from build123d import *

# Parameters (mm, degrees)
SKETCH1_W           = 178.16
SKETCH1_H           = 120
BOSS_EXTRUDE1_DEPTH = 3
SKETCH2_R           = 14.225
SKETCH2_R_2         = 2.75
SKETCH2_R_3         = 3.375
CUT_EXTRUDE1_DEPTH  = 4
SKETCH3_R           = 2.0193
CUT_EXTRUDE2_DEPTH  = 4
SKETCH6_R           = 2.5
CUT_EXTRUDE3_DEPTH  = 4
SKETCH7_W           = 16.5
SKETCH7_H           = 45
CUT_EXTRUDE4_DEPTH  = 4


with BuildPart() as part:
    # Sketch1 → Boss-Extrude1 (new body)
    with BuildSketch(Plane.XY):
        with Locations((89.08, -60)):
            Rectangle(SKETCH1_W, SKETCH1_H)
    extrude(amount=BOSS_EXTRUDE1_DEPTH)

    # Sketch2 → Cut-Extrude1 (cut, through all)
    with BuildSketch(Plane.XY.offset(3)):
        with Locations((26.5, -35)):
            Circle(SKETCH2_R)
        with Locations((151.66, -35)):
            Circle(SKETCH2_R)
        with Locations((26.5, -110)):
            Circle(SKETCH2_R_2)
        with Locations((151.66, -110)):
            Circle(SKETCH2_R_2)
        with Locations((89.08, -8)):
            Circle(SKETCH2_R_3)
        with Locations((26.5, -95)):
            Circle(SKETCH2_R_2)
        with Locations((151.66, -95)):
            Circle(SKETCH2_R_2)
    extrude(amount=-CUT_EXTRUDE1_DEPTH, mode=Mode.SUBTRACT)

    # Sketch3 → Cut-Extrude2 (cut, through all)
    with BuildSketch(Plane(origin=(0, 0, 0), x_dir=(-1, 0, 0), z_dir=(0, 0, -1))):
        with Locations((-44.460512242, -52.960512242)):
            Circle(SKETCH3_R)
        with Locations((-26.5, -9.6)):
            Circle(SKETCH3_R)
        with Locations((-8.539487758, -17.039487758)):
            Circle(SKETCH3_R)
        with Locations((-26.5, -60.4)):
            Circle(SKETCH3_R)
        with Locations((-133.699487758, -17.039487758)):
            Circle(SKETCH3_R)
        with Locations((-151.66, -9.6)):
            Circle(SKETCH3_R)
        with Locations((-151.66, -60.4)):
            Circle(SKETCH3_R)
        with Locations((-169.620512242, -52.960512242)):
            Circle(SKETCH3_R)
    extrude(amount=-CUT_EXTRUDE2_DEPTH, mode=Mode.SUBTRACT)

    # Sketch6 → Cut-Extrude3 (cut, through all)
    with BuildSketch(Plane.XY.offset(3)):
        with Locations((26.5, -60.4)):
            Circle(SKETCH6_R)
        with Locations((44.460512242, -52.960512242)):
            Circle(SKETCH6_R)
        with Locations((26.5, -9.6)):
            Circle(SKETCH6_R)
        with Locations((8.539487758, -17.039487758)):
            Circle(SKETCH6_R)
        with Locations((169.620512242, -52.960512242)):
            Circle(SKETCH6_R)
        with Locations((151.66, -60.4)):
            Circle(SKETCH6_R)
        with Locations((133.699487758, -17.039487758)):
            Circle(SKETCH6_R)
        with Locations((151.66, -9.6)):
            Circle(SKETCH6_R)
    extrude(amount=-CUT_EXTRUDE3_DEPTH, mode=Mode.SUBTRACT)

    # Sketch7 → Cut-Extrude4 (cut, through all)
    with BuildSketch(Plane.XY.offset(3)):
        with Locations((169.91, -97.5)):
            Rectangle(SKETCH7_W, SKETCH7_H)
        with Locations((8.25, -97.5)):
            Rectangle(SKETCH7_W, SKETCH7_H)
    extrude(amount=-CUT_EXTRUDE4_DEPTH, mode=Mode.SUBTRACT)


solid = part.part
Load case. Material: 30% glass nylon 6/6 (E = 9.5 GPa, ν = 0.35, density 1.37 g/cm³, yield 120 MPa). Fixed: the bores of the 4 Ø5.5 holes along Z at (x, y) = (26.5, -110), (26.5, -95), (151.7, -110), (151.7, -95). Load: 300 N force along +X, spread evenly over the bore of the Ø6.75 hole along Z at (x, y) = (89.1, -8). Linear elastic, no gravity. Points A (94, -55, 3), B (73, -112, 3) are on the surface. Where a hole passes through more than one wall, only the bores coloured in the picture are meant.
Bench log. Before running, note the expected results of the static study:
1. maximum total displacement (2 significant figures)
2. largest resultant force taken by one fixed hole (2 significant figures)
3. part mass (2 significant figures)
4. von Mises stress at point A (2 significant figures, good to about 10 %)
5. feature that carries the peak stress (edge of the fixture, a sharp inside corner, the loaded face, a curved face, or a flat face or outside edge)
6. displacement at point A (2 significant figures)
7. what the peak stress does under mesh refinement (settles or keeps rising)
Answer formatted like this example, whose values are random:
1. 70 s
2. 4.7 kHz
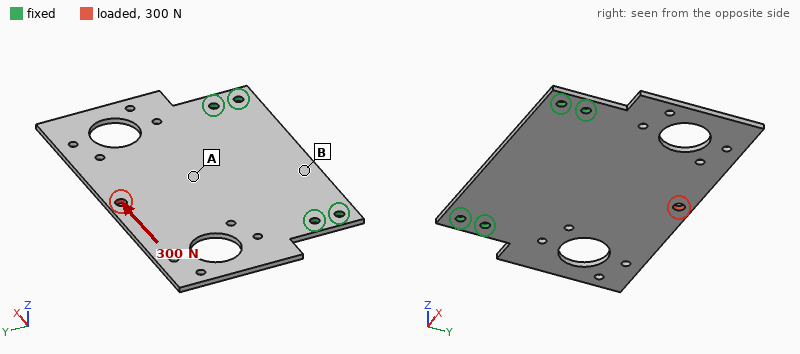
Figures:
1. 43 µm
2. 190 N
3. 75 g
4. 1.4 MPa
5. edge of the fixture
6. 15 µm
7. keeps rising
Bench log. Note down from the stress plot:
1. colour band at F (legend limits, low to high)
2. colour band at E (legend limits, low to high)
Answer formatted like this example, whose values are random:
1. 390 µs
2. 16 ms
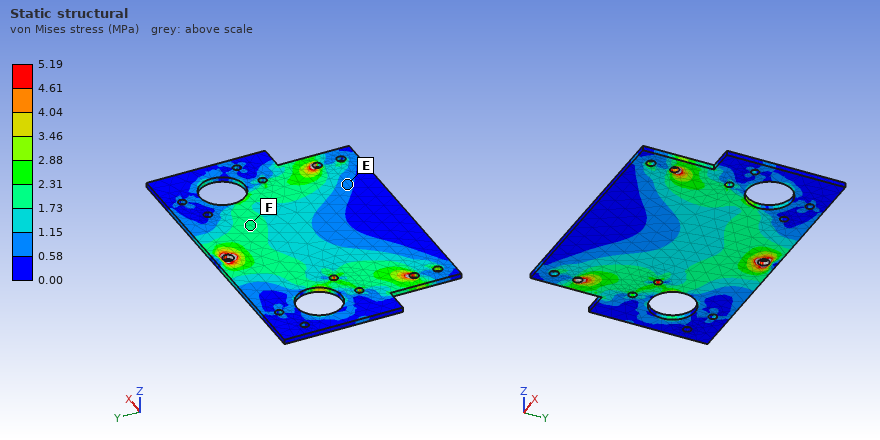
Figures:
1. 1.73 to 2.31 MPa
2. 0.58 to 1.15 MPa
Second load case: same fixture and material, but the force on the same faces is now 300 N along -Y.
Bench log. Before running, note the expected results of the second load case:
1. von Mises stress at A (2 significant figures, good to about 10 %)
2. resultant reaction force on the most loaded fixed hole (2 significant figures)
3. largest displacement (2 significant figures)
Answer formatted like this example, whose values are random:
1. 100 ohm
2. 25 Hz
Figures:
1. 0.99 MPa
2. 110 N
3. 28 µm
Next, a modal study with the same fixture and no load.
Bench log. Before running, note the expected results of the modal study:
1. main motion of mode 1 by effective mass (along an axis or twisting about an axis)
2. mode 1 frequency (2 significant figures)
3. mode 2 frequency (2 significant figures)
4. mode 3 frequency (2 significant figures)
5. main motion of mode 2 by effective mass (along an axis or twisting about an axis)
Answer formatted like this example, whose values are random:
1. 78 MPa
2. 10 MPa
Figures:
1. along Z
2. 110 Hz
3. 210 Hz
4. 370 Hz
5. twisting about Y
